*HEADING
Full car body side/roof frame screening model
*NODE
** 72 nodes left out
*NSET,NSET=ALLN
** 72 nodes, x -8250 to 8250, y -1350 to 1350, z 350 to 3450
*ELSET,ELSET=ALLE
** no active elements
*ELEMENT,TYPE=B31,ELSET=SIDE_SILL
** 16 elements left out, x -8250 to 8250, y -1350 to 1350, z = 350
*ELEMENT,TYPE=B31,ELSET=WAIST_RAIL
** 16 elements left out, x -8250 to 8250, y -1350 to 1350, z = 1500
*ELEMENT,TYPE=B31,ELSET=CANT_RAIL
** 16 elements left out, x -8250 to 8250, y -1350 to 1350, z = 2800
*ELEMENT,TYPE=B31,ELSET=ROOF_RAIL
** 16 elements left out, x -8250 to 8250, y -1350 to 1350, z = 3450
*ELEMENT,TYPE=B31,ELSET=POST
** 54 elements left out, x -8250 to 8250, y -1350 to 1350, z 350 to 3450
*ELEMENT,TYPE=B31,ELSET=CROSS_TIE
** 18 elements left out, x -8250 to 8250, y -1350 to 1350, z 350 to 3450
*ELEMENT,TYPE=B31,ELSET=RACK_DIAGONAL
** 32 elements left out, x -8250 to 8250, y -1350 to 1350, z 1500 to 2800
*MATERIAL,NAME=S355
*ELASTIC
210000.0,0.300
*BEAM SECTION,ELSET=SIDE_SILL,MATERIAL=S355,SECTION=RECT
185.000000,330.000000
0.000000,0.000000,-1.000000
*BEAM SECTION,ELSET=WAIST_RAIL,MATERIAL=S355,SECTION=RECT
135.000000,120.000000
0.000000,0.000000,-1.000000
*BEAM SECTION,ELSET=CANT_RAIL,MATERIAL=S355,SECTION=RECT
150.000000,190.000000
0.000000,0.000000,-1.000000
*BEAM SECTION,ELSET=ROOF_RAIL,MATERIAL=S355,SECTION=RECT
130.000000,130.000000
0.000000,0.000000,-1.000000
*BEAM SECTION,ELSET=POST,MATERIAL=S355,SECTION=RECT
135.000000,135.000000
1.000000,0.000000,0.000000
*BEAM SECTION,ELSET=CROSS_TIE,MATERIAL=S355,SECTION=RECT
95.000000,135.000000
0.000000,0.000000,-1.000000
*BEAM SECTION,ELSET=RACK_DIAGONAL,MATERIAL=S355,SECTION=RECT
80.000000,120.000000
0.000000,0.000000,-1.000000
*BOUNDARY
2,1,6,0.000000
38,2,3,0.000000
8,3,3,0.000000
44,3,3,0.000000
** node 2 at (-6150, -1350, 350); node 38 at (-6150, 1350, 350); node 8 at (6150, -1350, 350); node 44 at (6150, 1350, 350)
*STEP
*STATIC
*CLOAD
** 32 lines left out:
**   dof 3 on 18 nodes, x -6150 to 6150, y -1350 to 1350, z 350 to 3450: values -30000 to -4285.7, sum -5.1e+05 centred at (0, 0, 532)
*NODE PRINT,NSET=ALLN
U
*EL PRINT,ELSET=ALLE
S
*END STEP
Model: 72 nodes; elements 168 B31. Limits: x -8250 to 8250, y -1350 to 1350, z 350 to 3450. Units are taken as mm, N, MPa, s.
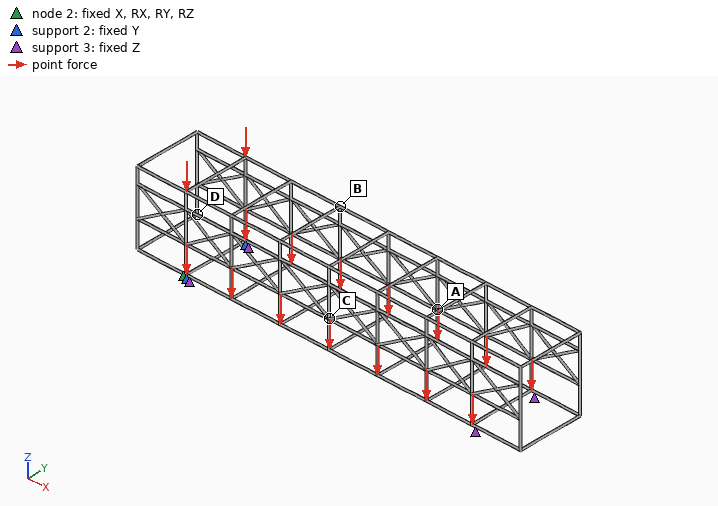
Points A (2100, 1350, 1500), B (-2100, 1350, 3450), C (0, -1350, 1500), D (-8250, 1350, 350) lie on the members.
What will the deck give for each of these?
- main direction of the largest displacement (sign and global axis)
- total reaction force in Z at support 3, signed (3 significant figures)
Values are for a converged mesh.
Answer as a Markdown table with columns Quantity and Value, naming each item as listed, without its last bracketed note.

| Quantity | Value |
|---|---|
| main direction of the largest displacement | -Z |
| total reaction force in Z at support 3, signed | 5.10e+05 N |
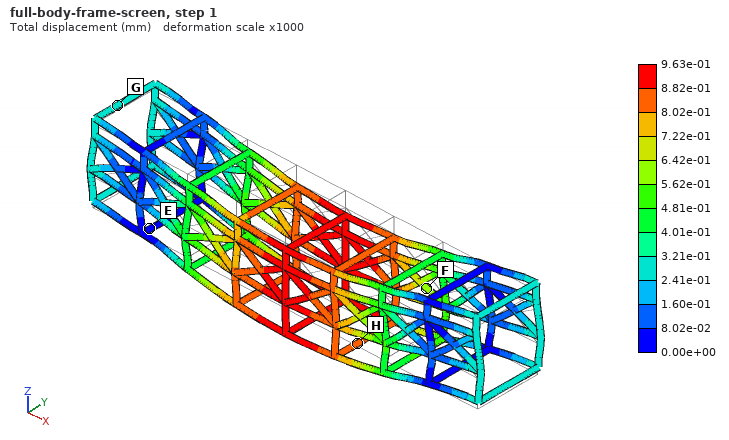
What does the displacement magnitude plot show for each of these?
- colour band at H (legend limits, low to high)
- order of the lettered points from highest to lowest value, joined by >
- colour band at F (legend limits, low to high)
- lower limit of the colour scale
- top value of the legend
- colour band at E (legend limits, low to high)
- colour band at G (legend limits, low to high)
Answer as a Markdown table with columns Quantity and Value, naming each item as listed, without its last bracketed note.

| Quantity | Value |
|---|---|
| colour band at H | 8.02e-01 to 8.82e-01 mm |
| order of the lettered points from highest to lowest value, joined by > | H > F > G > E |
| colour band at F | 5.62e-01 to 6.42e-01 mm |
| lower limit of the colour scale | 0.00e+00 mm |
| top value of the legend | 9.63e-01 mm |
| colour band at E | 0.00e+00 to 8.02e-02 mm |
| colour band at G | 2.41e-01 to 3.21e-01 mm |
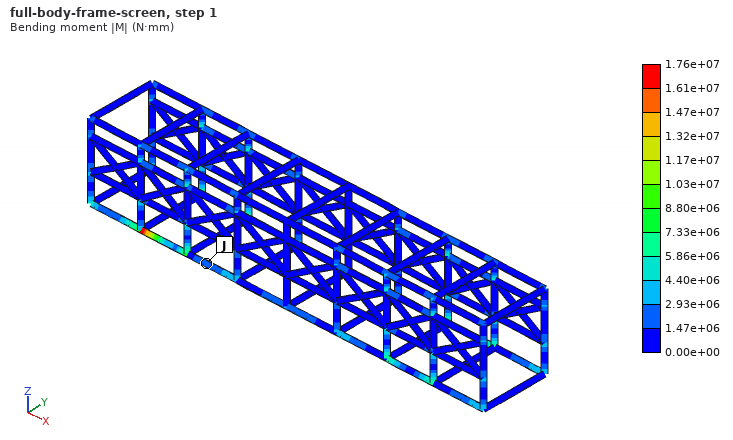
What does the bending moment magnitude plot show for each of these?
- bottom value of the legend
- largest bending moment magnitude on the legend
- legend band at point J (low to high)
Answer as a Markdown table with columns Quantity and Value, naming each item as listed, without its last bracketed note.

| Quantity | Value |
|---|---|
| bottom value of the legend | 0.00e+00 N·mm |
| largest bending moment magnitude on the legend | 1.76e+07 N·mm |
| legend band at point J | 1.47e+06 to 2.93e+06 N·mm |
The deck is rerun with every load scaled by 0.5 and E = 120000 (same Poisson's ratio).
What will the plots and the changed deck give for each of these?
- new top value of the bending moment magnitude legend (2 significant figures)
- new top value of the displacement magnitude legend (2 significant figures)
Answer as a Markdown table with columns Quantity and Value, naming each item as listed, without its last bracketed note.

| Quantity | Value |
|---|---|
| new top value of the bending moment magnitude legend | 8.8e+06 N·mm |
| new top value of the displacement magnitude legend | 0.84 mm |
